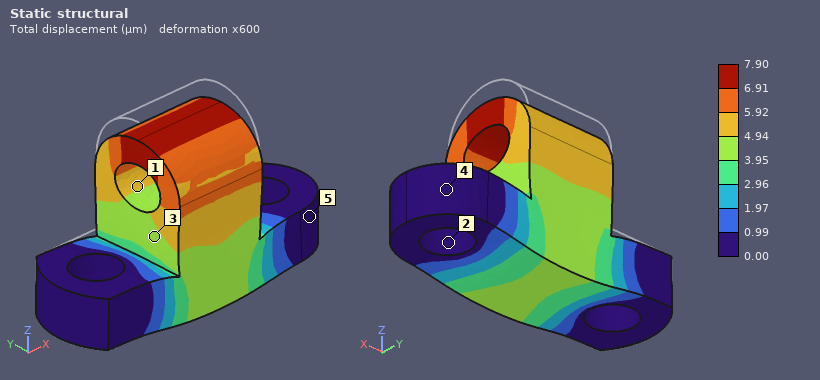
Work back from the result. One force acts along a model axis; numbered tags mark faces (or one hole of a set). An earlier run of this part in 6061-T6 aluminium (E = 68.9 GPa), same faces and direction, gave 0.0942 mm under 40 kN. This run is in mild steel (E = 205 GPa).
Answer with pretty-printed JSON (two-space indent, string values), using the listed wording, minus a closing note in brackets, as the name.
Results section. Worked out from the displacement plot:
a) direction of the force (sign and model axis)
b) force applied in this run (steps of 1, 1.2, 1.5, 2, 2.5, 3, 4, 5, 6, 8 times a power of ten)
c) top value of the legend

{
  "direction of the force": "-Z",
  "force applied in this run": "10 kN",
  "top value of the legend": "7.90 µm"
}
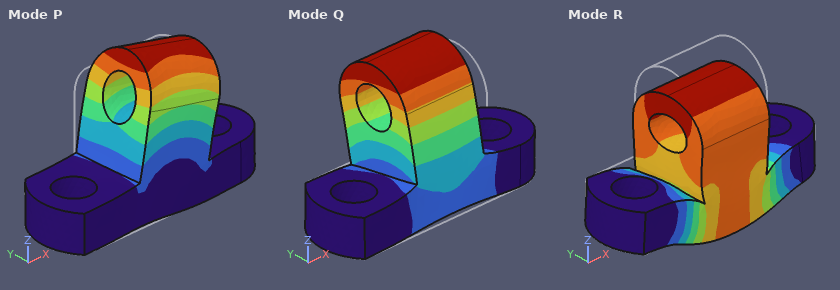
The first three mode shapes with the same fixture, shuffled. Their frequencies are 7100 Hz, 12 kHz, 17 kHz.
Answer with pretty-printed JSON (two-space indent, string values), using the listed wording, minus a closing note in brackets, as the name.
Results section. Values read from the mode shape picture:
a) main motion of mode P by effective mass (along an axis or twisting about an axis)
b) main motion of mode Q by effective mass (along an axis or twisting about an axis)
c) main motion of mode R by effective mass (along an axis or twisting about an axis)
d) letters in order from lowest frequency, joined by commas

{
  "main motion of mode P by effective mass": "along X",
  "main motion of mode Q by effective mass": "along Y",
  "main motion of mode R by effective mass": "along Z",
  "letters in order from lowest frequency, joined by commas": "Q, P, R"
}
